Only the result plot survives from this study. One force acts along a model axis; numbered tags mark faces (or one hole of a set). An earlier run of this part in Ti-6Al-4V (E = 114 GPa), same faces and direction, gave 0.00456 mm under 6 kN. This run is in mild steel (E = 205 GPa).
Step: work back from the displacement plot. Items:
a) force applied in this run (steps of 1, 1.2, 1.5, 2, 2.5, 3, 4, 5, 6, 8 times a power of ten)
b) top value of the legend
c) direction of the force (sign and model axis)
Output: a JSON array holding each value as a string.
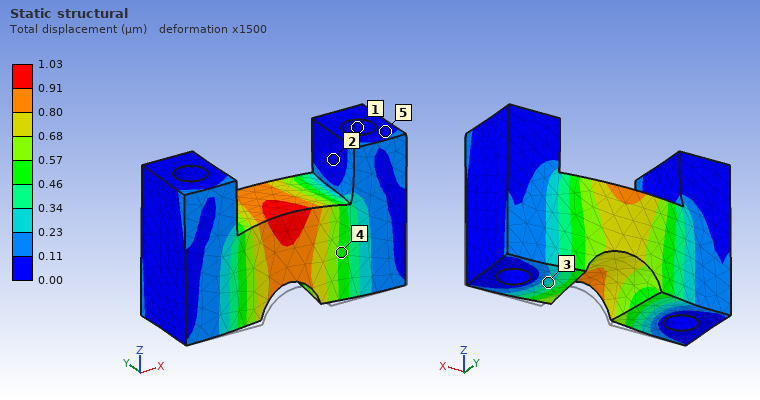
["2.5 kN", "1.03 µm", "+Y"]
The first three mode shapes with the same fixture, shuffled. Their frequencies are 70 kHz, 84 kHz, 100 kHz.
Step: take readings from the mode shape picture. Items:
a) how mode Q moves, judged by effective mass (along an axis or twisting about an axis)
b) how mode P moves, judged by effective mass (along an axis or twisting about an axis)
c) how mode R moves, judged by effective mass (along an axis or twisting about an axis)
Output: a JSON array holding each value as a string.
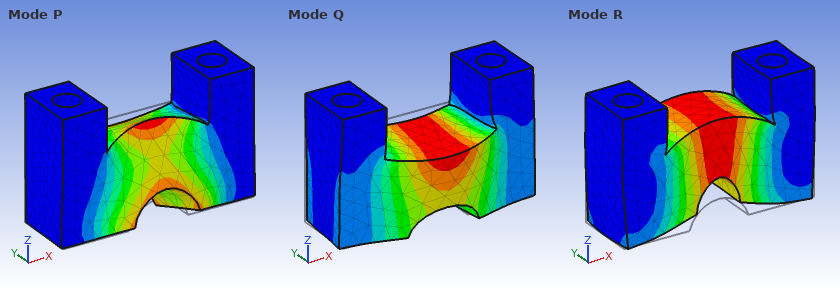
["along Y", "twisting about X", "along Z"]
